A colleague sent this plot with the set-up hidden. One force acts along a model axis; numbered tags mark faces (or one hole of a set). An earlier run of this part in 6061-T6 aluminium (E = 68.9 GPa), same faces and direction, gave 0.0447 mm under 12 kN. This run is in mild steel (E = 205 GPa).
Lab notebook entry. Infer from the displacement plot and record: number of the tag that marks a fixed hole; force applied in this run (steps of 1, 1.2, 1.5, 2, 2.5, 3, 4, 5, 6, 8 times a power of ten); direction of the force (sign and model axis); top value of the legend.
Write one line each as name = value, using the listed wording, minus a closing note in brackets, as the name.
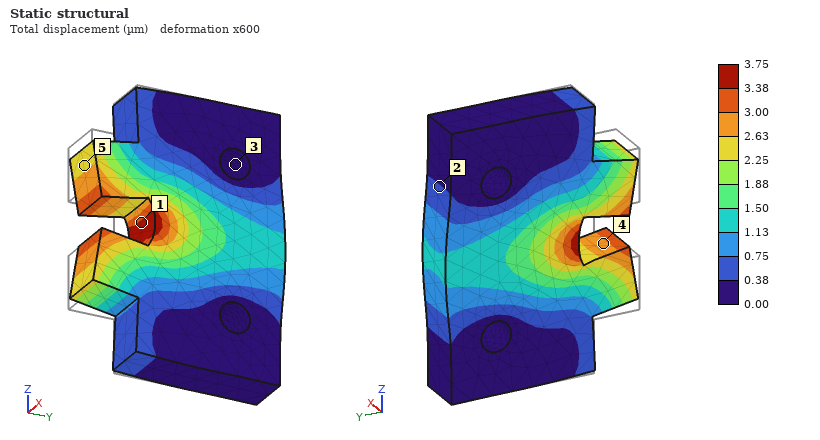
number of the tag that marks a fixed hole = 3
force applied in this run = 3 kN
direction of the force = +Y
top value of the legend = 3.75 µm
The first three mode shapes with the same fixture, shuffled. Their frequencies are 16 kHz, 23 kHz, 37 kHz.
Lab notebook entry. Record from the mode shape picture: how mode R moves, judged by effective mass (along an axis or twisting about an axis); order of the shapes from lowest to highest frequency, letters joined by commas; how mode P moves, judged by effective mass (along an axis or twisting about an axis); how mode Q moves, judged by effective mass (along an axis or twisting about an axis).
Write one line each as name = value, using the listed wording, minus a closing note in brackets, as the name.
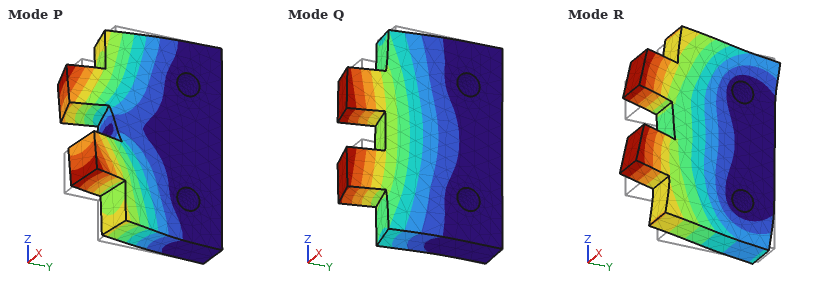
how mode R moves, judged by effective mass = along Z
order of the shapes from lowest to highest frequency, letters joined by commas = Q, P, R
how mode P moves, judged by effective mass = twisting about Y
how mode Q moves, judged by effective mass = along X
